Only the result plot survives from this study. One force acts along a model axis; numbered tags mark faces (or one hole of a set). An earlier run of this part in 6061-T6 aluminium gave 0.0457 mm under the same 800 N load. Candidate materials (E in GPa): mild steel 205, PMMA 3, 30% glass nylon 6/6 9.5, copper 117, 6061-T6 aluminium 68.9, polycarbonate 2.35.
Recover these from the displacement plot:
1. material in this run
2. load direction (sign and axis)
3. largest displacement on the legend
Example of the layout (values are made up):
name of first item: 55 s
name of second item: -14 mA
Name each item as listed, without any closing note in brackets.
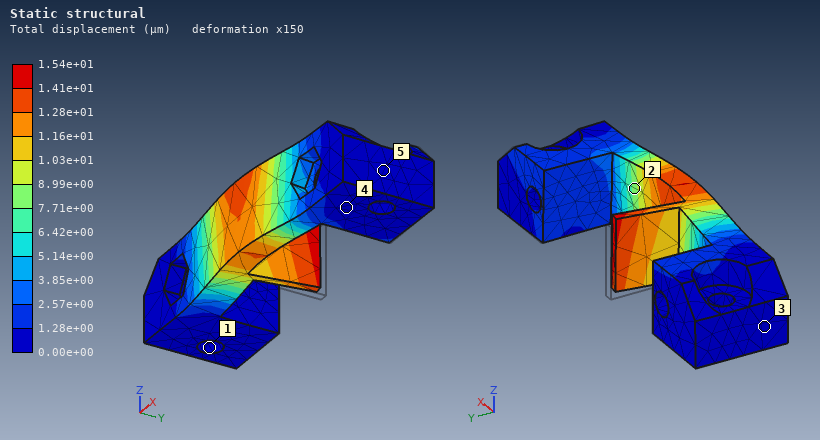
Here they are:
material in this run: mild steel
load direction: -Y
largest displacement on the legend: 1.54e+01 µm
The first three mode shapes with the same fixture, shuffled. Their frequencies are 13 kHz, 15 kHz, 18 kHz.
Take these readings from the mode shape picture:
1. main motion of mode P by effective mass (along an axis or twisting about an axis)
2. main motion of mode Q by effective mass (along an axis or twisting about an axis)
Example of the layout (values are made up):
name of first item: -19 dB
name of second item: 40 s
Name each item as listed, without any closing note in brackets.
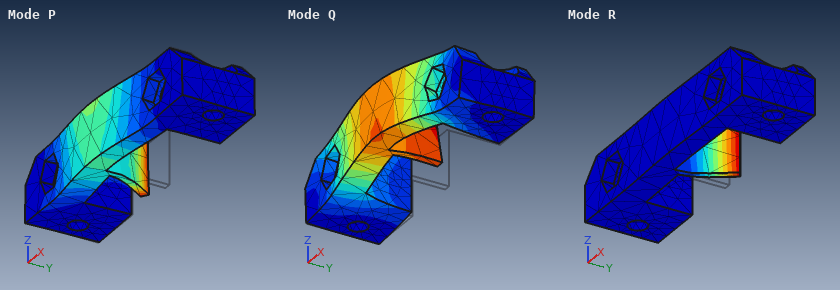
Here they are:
main motion of mode P by effective mass: along Y
main motion of mode Q by effective mass: along Z
